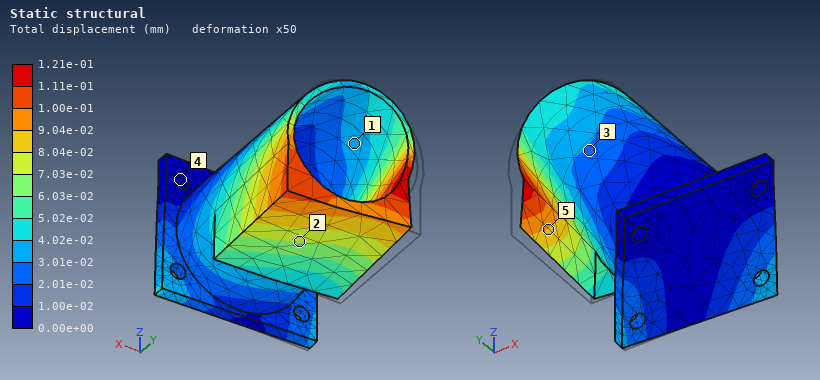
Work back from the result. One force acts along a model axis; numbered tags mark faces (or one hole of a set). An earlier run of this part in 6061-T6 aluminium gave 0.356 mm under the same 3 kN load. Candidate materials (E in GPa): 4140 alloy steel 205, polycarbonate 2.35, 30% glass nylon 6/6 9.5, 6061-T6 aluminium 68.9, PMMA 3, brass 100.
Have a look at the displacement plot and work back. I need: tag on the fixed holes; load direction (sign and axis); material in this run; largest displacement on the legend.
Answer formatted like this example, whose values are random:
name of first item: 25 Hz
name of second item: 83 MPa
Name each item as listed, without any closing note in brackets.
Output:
tag on the fixed holes: 4
load direction: +X
material in this run: 4140 alloy steel
largest displacement on the legend: 1.21e-01 mm
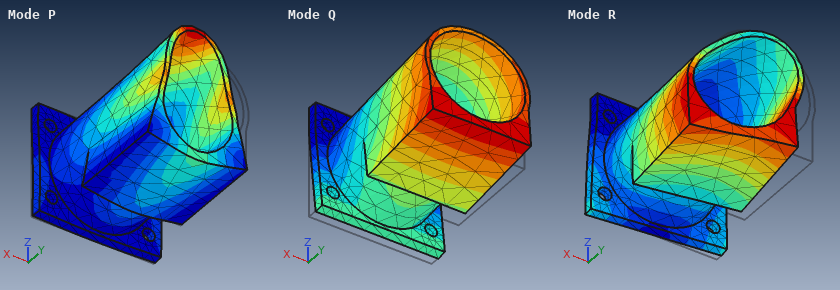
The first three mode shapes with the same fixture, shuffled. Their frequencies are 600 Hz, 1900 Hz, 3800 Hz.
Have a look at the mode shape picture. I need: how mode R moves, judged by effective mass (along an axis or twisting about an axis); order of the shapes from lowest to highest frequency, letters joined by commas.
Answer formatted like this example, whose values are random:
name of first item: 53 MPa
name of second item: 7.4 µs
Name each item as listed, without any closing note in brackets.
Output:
how mode R moves, judged by effective mass: along X
order of the shapes from lowest to highest frequency, letters joined by commas: Q, R, P
